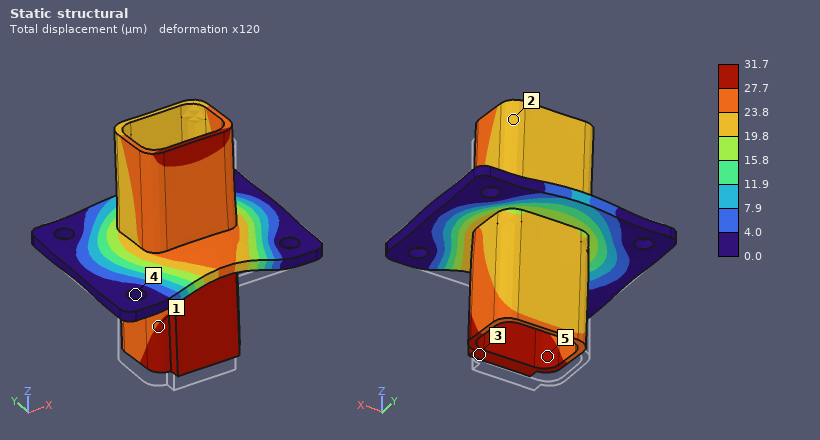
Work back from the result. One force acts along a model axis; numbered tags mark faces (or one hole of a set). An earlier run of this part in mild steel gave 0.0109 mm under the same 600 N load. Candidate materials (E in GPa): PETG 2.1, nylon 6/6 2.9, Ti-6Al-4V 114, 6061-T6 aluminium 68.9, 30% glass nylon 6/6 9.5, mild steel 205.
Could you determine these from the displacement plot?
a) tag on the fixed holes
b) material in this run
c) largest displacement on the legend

4
6061-T6 aluminium
31.7 µm
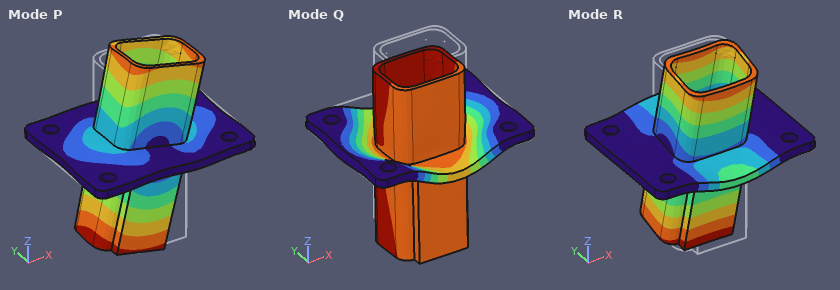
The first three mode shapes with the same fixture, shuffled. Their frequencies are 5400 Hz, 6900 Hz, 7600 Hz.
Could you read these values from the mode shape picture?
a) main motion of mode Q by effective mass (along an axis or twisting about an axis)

along Z
